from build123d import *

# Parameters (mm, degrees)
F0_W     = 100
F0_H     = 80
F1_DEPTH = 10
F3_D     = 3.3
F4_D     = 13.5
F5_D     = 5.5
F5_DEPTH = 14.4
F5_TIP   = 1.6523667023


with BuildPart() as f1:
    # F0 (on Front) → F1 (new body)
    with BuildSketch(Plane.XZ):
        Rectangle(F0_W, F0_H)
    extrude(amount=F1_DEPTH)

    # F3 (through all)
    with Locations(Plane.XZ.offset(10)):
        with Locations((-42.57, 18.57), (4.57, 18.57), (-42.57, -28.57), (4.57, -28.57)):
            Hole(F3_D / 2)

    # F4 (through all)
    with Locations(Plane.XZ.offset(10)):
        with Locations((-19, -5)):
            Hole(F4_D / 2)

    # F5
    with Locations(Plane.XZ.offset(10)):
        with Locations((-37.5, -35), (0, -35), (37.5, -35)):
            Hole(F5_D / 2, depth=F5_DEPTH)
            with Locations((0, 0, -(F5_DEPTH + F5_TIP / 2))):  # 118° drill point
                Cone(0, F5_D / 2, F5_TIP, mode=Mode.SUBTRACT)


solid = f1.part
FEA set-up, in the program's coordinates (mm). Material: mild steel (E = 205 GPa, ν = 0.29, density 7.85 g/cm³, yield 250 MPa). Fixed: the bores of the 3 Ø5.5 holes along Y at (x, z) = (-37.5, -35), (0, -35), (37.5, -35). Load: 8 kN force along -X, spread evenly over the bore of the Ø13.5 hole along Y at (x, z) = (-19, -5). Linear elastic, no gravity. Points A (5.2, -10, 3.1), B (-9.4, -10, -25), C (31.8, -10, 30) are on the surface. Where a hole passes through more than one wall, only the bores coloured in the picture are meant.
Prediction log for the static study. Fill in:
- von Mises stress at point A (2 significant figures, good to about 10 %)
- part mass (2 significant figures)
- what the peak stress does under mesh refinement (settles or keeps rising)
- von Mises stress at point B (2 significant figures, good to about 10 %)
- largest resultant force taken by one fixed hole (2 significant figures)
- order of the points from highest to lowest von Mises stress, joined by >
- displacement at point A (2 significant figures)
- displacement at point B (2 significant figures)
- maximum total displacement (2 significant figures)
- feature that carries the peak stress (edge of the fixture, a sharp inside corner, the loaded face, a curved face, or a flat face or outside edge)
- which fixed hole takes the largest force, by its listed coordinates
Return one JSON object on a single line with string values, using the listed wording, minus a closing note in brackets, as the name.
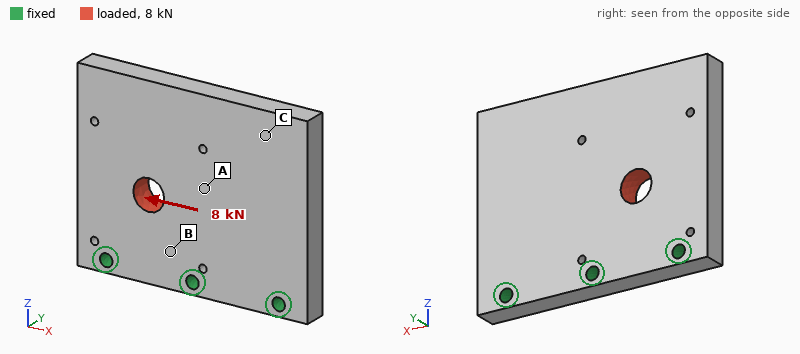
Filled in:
{"von Mises stress at point A": "11 MPa", "part mass": "610 g", "what the peak stress does under mesh refinement": "keeps rising", "von Mises stress at point B": "20 MPa", "largest resultant force taken by one fixed hole": "4.1 kN", "order of the points from highest to lowest von Mises stress, joined by >": "B > A > C", "displacement at point A": "4.9 µm", "displacement at point B": "1.8 µm", "maximum total displacement": "7.4 µm", "feature that carries the peak stress": "edge of the fixture", "which fixed hole takes the largest force, by its listed coordinates": "(-37.5, -35)"}
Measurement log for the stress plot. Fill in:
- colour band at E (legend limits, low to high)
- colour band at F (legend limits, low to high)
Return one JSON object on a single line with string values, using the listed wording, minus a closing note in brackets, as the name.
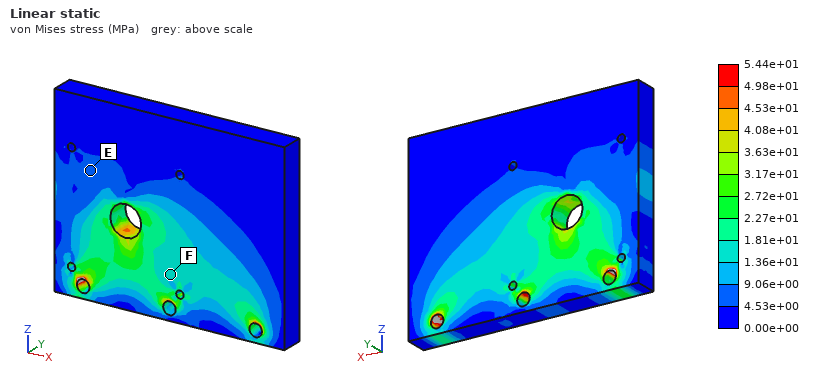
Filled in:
{"colour band at E": "4.53e+00 to 9.06e+00 MPa", "colour band at F": "1.36e+01 to 1.81e+01 MPa"}
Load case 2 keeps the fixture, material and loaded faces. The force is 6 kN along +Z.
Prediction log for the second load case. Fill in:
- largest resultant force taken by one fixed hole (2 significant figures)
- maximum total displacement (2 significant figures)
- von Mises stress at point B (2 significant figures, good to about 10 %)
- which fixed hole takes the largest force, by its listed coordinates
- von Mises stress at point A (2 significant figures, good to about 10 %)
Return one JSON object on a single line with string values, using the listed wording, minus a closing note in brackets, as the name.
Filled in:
{"largest resultant force taken by one fixed hole": "3.4 kN", "maximum total displacement": "3.1 µm", "von Mises stress at point B": "11 MPa", "which fixed hole takes the largest force, by its listed coordinates": "(-37.5, -35)", "von Mises stress at point A": "3.4 MPa"}
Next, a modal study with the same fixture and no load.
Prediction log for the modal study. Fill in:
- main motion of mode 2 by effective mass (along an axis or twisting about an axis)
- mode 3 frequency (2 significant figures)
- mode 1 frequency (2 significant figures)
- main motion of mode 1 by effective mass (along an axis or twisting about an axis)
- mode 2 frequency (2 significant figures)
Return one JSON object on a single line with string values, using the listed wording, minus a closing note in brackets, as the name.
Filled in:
{"main motion of mode 2 by effective mass": "twisting about Z", "mode 3 frequency": "6600 Hz", "mode 1 frequency": "1300 Hz", "main motion of mode 1 by effective mass": "along Y", "mode 2 frequency": "2700 Hz"}
